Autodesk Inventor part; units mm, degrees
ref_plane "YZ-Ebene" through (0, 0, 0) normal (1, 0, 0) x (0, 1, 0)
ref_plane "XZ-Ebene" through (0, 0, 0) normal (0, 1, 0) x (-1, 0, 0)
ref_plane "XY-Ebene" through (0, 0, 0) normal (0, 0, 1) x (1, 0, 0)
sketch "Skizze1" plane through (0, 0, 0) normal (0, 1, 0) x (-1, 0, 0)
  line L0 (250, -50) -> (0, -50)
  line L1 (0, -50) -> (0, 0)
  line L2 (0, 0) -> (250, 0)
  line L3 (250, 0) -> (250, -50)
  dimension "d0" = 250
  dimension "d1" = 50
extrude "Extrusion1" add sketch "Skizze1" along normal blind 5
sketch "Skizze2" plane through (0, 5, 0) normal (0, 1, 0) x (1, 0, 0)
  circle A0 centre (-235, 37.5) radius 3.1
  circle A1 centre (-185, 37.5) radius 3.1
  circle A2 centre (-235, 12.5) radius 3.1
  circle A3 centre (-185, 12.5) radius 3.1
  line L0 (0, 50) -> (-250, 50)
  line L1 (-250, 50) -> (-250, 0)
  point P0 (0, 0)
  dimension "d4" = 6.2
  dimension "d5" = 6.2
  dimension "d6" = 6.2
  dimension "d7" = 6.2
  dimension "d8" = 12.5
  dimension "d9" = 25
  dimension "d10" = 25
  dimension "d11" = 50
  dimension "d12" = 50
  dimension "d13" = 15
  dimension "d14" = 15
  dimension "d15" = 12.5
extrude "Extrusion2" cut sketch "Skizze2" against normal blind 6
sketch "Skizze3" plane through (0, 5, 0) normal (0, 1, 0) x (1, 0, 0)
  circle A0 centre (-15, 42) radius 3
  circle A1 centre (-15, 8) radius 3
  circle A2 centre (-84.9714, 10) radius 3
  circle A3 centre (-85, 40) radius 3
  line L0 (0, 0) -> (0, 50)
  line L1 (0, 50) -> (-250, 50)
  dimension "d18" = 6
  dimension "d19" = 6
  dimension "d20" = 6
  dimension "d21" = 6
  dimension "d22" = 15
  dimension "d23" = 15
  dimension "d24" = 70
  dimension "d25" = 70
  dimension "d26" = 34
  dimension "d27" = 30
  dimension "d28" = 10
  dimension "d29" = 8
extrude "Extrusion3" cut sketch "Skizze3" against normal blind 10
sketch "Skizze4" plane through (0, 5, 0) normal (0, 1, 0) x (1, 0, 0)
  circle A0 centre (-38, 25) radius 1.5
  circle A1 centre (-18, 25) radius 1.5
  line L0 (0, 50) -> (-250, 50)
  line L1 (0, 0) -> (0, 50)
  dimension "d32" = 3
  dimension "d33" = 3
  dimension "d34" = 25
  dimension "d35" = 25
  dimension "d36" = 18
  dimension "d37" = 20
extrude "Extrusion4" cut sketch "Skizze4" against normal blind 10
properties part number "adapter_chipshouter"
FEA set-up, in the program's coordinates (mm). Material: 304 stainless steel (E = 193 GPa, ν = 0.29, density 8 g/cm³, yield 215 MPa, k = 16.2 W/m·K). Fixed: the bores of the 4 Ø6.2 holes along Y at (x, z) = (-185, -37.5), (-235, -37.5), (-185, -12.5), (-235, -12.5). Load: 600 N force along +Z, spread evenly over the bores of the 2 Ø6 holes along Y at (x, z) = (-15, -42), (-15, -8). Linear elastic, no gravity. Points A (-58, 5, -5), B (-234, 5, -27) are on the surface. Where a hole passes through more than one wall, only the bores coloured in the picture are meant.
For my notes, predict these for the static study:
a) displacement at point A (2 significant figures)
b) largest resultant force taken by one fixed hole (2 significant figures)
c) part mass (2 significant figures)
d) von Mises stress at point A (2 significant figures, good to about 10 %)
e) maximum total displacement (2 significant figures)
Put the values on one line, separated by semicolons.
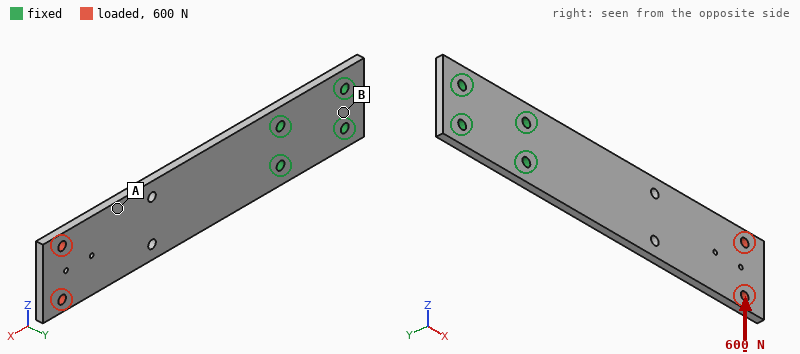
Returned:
0.075 mm; 2.9 kN; 490 g; 10 MPa; 0.13 mm
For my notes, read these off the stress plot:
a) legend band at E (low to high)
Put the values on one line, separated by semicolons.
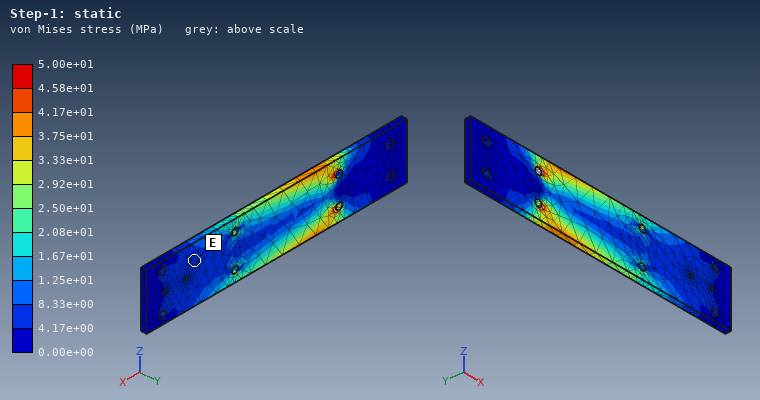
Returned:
4.17e+00 to 8.33e+00 MPa
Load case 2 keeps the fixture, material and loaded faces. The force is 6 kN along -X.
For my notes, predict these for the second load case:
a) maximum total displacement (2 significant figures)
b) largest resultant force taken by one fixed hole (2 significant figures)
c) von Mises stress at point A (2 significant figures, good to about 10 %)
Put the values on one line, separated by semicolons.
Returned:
24 µm; 2.8 kN; 24 MPa
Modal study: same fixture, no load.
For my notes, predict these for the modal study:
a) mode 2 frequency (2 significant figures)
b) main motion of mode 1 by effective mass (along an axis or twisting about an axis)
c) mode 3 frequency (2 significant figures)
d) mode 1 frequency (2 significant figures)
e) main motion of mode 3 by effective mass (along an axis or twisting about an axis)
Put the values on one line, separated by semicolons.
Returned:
730 Hz; along Y; 860 Hz; 120 Hz; twisting about X
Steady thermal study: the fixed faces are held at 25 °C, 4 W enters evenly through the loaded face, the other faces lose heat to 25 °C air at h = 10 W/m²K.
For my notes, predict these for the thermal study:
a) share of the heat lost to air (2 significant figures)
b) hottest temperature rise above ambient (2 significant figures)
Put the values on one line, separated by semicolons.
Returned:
91 %; 51 K
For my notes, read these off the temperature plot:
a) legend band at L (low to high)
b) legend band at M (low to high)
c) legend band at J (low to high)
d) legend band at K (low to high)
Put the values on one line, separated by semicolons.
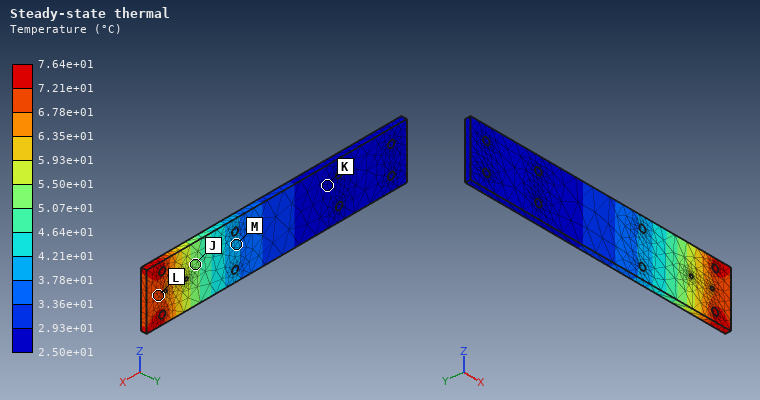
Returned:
6.78e+01 to 7.21e+01 °C; 3.78e+01 to 4.21e+01 °C; 5.07e+01 to 5.50e+01 °C; 2.50e+01 to 2.93e+01 °C
